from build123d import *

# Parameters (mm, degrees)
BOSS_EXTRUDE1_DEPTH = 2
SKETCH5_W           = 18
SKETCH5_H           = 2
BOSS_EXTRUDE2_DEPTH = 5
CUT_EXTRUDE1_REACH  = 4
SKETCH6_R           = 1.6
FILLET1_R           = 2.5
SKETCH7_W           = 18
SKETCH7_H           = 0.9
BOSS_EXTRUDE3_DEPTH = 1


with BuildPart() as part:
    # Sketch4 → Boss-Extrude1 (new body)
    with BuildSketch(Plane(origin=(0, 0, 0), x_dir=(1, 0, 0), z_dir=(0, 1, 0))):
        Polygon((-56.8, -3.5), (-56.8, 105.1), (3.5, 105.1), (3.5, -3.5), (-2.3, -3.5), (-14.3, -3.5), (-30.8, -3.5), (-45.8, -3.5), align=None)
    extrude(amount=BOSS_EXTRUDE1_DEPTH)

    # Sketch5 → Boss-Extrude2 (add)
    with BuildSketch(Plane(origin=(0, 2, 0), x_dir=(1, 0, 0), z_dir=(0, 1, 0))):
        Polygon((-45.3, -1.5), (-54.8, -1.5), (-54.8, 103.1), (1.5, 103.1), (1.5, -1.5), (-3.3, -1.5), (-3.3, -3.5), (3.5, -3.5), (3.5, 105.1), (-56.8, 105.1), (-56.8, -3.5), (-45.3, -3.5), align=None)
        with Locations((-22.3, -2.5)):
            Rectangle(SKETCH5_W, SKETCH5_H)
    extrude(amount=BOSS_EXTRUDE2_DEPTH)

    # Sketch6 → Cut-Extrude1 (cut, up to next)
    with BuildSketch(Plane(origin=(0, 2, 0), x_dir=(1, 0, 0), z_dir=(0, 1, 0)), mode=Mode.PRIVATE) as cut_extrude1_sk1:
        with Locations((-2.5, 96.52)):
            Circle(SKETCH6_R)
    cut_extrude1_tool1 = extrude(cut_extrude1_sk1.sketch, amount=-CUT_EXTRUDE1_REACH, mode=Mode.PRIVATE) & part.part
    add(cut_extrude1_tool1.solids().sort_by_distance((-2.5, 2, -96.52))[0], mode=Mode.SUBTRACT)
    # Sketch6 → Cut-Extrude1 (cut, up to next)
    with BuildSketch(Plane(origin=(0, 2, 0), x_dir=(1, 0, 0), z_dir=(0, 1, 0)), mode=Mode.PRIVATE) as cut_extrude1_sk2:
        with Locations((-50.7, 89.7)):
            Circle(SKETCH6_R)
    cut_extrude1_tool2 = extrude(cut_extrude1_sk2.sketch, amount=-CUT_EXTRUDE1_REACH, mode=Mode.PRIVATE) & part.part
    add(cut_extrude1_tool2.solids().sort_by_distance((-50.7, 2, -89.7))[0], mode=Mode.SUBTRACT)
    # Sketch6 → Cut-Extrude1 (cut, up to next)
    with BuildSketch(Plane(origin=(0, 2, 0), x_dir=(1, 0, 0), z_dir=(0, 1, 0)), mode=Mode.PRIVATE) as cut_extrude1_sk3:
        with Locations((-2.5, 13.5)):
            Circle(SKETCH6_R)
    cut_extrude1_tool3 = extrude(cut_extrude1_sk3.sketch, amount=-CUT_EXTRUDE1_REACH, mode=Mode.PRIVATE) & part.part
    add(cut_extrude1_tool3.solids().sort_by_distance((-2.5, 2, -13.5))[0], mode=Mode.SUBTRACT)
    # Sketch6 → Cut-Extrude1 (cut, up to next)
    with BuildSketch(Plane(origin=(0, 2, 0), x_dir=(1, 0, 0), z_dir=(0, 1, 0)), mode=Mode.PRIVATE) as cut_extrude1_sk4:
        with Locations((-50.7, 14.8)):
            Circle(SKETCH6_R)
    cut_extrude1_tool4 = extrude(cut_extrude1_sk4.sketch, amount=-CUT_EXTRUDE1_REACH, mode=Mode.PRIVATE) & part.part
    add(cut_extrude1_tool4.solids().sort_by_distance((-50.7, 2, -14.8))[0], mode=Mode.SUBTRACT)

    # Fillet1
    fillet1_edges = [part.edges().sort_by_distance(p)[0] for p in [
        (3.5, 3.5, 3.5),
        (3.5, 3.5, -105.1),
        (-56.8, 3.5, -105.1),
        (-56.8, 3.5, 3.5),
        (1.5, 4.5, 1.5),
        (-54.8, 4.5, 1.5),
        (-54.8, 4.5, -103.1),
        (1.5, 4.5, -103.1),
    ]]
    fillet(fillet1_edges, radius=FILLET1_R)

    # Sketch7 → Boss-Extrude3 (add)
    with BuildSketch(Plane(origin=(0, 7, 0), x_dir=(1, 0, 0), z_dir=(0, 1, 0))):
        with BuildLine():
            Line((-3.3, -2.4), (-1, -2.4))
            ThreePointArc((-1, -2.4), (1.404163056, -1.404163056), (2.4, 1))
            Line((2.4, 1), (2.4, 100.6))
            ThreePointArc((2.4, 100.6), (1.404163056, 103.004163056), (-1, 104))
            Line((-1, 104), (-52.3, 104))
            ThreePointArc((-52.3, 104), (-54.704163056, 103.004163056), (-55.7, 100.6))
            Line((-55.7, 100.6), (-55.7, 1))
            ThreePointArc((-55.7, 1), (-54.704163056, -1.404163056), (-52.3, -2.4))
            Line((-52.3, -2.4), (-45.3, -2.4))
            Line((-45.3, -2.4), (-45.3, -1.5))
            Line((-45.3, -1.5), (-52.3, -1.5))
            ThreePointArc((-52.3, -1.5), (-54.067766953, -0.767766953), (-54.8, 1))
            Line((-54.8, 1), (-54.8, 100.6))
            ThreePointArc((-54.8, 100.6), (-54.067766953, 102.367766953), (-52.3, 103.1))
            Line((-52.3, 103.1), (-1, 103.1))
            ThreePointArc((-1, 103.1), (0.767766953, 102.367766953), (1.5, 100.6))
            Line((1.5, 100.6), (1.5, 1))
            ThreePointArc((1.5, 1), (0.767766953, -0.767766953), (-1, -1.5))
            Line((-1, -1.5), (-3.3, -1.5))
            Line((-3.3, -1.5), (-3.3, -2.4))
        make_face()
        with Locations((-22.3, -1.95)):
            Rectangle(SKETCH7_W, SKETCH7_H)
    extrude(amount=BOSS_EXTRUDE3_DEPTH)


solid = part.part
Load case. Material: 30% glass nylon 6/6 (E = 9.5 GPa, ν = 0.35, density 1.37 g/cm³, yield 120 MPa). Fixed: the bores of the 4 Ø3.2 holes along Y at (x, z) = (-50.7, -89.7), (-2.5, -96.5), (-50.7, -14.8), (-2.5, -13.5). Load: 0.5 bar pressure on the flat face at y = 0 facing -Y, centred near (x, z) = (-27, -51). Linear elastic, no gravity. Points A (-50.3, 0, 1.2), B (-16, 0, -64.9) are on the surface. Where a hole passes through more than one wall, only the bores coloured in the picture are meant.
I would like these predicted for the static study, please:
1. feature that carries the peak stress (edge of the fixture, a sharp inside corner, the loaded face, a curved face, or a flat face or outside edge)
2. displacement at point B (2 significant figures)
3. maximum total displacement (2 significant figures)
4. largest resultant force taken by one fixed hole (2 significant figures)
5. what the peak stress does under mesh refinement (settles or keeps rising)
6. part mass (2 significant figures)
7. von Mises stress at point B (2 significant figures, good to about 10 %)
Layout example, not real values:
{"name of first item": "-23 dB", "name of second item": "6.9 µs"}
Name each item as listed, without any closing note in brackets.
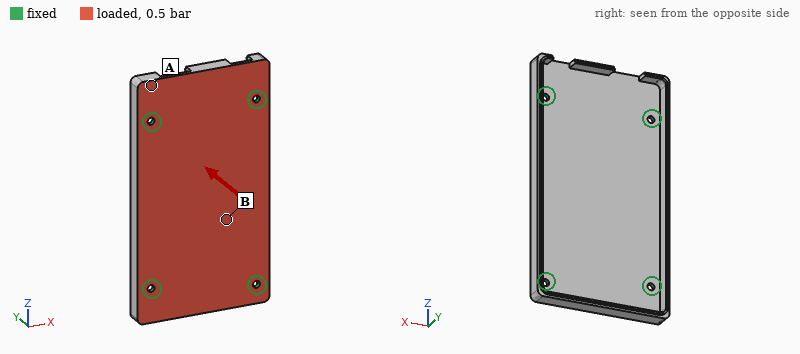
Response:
{"feature that carries the peak stress": "edge of the fixture", "displacement at point B": "0.46 mm", "maximum total displacement": "0.55 mm", "largest resultant force taken by one fixed hole": "96 N", "what the peak stress does under mesh refinement": "keeps rising", "part mass": "22 g", "von Mises stress at point B": "12 MPa"}
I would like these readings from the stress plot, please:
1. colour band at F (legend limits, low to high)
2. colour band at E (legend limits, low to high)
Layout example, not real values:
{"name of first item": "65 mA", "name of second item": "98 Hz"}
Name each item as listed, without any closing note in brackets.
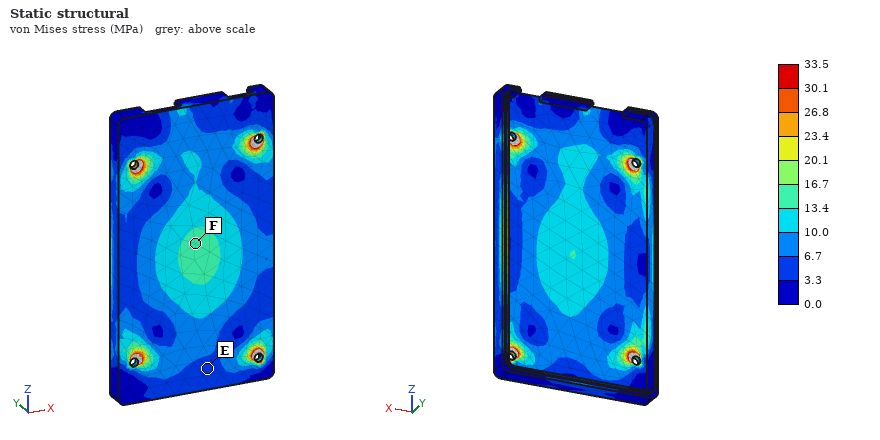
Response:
{"colour band at F": "13.4 to 16.7 MPa", "colour band at E": "3.3 to 6.7 MPa"}
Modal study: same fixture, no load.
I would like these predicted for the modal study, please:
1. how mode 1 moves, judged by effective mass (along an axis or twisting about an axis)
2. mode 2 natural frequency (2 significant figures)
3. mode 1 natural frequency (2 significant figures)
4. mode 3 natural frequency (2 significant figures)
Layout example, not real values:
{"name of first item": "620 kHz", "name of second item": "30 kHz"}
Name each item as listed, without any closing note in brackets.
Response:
{"how mode 1 moves, judged by effective mass": "along Y", "mode 2 natural frequency": "1800 Hz", "mode 1 natural frequency": "1100 Hz", "mode 3 natural frequency": "1900 Hz"}
